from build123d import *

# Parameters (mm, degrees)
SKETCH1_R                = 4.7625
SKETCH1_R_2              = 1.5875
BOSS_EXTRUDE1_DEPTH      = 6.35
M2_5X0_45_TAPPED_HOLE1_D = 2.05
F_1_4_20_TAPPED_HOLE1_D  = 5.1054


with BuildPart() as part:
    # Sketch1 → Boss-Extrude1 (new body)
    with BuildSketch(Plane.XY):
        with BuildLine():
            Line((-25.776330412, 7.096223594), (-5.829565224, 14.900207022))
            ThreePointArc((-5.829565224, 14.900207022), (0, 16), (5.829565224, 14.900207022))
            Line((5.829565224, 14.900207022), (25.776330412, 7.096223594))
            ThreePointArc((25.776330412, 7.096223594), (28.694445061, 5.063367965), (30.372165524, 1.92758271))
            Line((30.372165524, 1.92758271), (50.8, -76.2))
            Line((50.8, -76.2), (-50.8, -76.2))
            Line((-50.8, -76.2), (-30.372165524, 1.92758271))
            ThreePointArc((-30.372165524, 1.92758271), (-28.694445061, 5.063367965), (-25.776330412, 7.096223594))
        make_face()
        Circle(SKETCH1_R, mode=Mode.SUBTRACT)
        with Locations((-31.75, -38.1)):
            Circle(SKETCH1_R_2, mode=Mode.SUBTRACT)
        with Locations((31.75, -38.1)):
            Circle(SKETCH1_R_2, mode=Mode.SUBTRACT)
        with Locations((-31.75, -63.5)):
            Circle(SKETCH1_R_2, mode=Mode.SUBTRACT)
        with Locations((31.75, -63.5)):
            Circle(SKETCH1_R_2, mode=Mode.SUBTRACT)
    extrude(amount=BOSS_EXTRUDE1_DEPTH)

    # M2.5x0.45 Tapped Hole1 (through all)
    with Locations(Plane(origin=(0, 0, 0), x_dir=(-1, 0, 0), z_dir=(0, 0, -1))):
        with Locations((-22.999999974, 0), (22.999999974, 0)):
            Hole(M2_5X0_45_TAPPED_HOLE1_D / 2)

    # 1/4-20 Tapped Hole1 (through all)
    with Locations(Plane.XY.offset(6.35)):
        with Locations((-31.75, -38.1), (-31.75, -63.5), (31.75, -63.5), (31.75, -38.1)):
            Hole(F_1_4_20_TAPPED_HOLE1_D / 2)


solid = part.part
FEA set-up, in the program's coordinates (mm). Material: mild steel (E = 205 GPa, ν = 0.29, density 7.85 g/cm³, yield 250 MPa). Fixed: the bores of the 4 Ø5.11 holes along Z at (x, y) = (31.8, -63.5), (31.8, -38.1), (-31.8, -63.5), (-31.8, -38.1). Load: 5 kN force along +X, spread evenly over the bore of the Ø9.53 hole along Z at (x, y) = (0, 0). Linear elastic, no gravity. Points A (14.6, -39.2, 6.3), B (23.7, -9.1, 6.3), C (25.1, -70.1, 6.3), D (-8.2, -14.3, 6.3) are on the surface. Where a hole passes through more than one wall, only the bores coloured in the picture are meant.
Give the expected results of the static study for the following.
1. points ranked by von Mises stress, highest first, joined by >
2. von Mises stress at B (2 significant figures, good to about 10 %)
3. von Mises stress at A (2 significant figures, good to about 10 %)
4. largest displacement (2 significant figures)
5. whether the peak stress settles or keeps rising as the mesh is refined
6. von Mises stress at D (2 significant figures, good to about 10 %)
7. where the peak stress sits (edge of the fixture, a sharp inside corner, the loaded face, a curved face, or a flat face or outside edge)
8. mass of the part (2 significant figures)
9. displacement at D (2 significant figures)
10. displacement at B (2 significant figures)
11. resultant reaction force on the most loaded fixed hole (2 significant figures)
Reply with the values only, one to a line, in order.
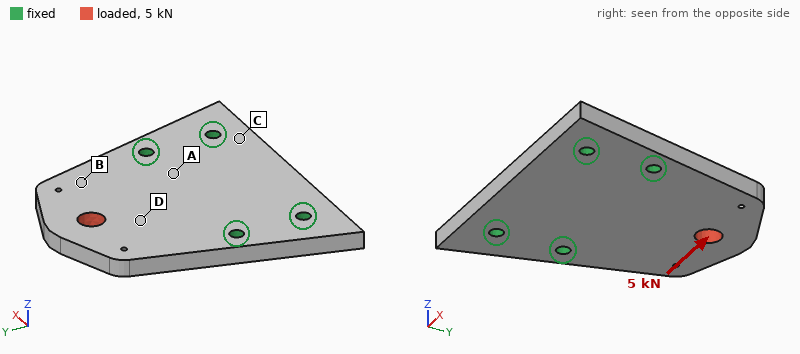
D > B > A > C
17 MPa
9.4 MPa
10 µm
keeps rising
24 MPa
edge of the fixture
340 g
4.9 µm
6.1 µm
3.4 kN
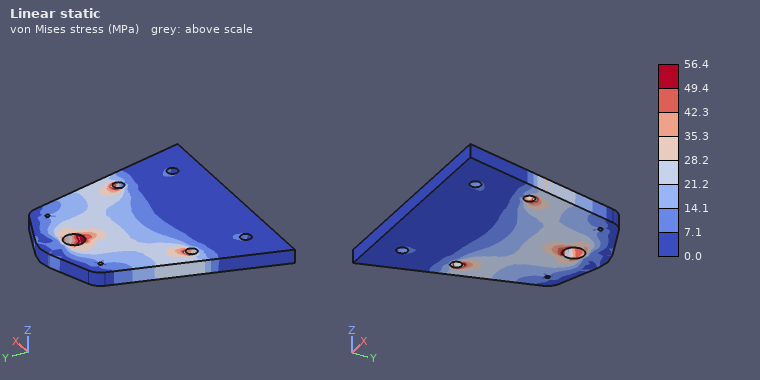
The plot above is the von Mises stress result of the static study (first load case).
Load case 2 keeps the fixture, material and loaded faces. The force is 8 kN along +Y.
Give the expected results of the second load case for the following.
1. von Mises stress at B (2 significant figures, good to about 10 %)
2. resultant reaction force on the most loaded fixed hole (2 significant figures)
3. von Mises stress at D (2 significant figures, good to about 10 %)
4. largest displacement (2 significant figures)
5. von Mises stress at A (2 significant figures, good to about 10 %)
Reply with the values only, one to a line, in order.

16 MPa
2.9 kN
29 MPa
9.2 µm
14 MPa
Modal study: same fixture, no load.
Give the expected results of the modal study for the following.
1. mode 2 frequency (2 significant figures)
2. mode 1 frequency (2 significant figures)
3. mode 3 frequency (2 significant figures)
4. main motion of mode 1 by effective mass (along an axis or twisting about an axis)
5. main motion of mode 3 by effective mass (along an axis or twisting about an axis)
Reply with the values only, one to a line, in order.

5200 Hz
2000 Hz
7600 Hz
along Z
along Z
